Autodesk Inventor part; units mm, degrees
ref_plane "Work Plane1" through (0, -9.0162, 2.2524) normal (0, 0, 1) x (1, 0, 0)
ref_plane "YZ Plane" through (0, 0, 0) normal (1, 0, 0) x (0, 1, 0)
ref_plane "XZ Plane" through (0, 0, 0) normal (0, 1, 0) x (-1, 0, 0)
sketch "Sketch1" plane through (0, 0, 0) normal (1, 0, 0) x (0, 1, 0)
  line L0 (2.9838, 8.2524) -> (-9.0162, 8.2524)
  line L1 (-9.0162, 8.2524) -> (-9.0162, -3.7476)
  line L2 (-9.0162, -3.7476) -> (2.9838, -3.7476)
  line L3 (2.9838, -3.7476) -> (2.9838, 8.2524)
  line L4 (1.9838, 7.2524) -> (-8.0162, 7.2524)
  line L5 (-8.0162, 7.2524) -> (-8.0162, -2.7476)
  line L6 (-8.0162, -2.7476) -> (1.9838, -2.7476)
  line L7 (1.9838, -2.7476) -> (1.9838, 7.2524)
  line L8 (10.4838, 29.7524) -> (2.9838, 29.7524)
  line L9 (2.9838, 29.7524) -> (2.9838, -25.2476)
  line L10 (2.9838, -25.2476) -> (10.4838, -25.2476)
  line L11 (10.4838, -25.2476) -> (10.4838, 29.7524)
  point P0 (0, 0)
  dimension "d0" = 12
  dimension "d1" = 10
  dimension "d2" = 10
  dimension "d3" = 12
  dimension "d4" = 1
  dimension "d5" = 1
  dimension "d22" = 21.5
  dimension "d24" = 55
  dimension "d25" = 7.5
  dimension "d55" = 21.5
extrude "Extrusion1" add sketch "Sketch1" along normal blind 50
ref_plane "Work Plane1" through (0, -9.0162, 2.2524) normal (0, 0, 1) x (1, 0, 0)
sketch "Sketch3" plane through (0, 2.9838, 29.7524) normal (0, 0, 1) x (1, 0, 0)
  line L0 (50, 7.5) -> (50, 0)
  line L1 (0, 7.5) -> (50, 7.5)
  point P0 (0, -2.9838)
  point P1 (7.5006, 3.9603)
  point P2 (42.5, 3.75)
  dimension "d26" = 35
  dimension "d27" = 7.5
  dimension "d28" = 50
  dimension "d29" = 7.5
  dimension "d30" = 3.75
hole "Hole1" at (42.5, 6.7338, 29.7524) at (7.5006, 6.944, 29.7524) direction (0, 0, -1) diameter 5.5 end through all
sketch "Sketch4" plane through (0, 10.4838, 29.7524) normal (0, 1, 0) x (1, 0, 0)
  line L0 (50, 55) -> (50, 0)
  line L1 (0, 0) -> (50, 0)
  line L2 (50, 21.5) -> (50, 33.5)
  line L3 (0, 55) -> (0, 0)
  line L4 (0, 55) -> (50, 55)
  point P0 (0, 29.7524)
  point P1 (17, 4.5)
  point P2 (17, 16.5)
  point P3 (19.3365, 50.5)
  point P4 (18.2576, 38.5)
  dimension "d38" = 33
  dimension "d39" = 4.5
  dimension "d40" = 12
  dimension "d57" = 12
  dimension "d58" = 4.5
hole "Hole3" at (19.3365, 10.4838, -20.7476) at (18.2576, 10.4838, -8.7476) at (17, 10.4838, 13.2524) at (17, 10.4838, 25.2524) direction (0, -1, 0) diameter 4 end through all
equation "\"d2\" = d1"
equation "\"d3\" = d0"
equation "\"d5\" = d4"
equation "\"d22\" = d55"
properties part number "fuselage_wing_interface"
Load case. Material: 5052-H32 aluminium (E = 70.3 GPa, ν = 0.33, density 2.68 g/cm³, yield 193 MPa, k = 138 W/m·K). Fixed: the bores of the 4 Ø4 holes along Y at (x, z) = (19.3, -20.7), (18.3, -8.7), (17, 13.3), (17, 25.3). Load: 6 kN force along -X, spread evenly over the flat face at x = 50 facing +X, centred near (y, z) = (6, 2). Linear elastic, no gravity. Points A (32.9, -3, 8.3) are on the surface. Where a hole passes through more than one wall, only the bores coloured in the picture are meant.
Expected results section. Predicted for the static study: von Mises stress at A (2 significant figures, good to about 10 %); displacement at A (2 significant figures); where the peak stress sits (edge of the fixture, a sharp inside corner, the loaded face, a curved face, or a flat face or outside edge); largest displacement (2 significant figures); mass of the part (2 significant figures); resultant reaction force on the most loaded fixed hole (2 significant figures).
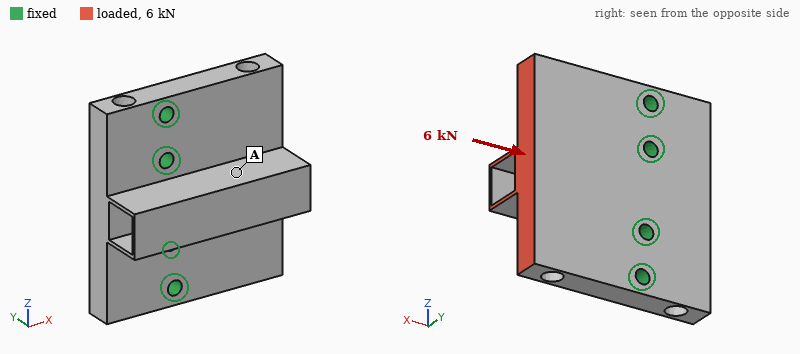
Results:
14 MPa
8.3 µm
a curved face
15 µm
53 g
1.7 kN
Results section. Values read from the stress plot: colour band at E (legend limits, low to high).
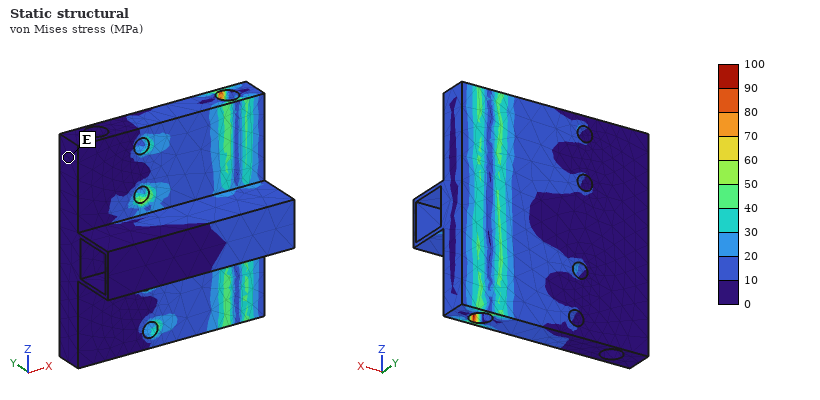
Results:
0 to 10 MPa
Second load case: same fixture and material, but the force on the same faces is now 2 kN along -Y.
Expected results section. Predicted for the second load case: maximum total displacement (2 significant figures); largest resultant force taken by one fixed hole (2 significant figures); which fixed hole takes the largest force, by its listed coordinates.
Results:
0.14 mm
820 N
(18.3, -8.7)
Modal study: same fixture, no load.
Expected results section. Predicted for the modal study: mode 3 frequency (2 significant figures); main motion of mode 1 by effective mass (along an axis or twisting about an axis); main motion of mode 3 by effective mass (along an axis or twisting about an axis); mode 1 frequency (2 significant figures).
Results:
11 kHz
along Y
twisting about X
6500 Hz
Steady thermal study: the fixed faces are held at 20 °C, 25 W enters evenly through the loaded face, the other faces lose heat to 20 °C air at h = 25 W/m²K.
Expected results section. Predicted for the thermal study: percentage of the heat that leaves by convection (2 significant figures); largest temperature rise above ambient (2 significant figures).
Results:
6.0 %
17 K
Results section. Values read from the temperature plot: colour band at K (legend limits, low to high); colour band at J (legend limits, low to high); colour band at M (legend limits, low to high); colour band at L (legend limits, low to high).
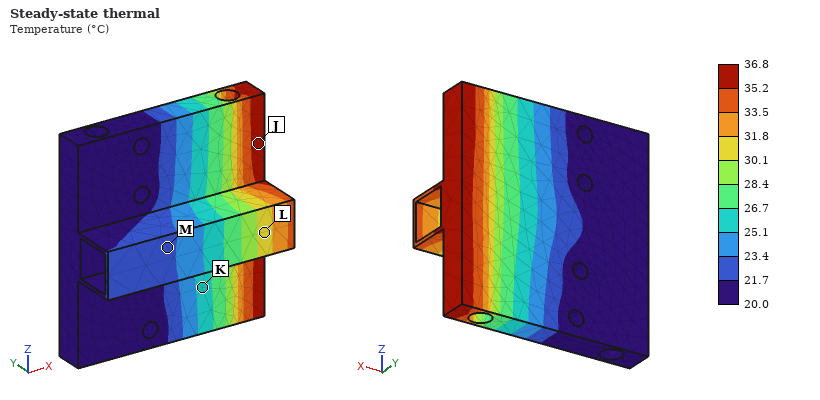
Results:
25.1 to 26.7 °C
35.2 to 36.8 °C
21.7 to 23.4 °C
30.1 to 31.8 °C
